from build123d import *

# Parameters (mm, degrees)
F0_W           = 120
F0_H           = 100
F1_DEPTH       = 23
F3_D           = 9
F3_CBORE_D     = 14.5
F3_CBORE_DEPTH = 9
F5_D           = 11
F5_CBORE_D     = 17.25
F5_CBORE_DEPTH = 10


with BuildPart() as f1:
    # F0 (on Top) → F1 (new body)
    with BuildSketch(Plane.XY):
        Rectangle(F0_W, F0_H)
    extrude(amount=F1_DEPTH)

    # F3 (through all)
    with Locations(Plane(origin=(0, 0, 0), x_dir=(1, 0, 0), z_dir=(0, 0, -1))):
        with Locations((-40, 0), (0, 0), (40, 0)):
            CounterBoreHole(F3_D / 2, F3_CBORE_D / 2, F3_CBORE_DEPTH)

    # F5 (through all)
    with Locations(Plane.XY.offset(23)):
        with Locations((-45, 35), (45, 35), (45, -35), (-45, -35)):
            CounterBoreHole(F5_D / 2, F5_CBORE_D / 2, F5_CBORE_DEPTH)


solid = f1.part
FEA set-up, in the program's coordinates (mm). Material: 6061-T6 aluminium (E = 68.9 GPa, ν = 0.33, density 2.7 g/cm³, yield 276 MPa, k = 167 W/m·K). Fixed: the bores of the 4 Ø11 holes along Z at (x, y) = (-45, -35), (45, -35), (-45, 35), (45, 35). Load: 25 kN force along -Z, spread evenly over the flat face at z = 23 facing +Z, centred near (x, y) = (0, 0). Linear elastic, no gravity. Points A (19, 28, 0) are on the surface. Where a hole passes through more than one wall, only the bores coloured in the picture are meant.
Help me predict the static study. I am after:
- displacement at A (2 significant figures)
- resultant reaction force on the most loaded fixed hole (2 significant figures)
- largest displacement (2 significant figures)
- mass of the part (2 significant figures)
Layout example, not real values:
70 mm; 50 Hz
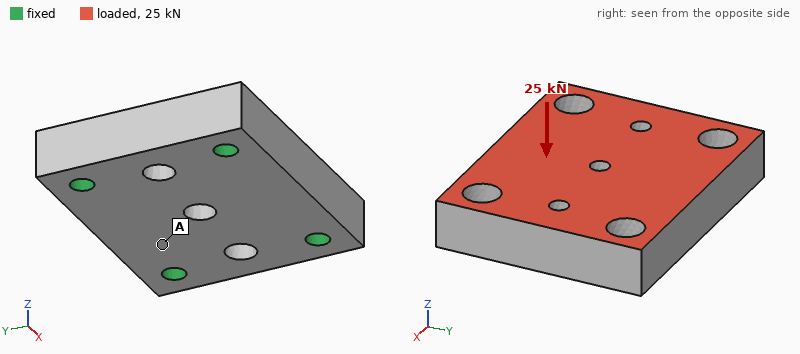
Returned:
14 µm; 6.8 kN; 20 µm; 690 g
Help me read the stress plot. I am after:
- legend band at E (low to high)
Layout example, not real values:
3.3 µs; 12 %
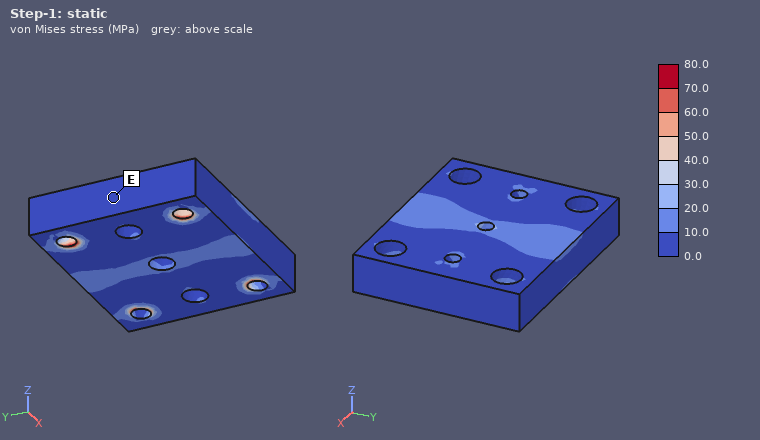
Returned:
0.0 to 10.0 MPa
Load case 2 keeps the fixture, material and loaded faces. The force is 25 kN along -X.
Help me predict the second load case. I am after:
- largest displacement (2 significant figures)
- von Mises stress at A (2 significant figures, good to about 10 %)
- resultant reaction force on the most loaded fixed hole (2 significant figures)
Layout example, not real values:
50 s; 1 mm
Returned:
11 µm; 6.1 MPa; 6.6 kN
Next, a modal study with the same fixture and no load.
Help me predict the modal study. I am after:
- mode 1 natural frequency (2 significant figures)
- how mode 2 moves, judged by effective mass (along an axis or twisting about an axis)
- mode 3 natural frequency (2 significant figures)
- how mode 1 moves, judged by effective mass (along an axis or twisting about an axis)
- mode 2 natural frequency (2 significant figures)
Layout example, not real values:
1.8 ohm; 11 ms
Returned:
8000 Hz; twisting about X; 13 kHz; along Z; 10 kHz
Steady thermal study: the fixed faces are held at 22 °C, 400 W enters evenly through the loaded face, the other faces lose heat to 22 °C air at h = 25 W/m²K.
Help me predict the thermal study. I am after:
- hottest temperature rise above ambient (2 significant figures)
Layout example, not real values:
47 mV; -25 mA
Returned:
18 K
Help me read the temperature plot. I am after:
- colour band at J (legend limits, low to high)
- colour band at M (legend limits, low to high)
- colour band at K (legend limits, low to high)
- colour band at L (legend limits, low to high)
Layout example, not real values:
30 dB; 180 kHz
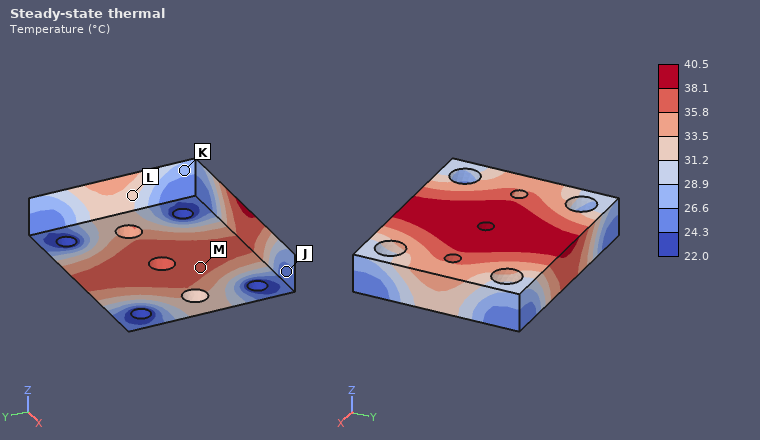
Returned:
24.3 to 26.6 °C; 35.8 to 38.1 °C; 26.6 to 28.9 °C; 31.2 to 33.5 °C
